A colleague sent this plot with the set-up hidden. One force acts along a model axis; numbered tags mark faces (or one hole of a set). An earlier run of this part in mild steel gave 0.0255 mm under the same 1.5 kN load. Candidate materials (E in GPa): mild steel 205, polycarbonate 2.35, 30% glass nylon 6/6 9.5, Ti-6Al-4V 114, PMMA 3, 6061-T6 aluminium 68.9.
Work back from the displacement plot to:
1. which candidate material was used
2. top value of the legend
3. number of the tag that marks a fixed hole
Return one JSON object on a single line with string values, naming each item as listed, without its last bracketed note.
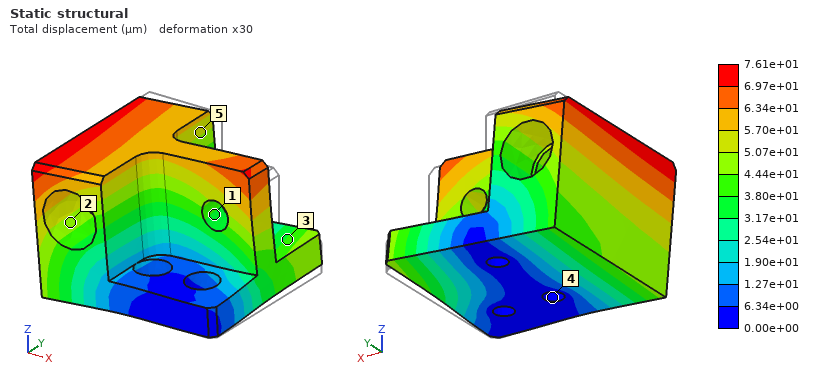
{"which candidate material was used": "6061-T6 aluminium", "top value of the legend": "7.61e+01 µm", "number of the tag that marks a fixed hole": "4"}
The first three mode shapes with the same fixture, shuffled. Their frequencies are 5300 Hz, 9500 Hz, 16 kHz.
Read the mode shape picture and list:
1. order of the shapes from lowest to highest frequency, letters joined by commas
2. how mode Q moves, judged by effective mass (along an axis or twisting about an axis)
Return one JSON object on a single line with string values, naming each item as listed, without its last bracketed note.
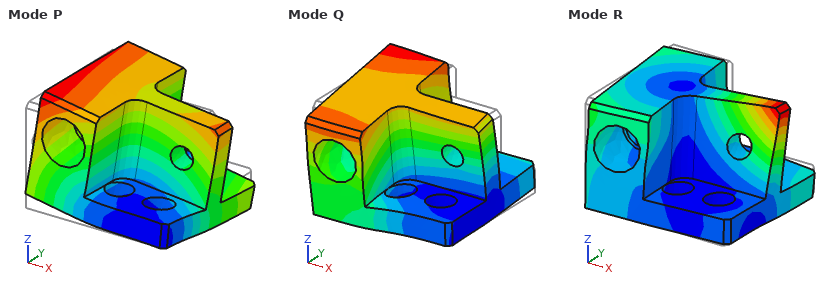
{"order of the shapes from lowest to highest frequency, letters joined by commas": "P, Q, R", "how mode Q moves, judged by effective mass": "along Y"}
